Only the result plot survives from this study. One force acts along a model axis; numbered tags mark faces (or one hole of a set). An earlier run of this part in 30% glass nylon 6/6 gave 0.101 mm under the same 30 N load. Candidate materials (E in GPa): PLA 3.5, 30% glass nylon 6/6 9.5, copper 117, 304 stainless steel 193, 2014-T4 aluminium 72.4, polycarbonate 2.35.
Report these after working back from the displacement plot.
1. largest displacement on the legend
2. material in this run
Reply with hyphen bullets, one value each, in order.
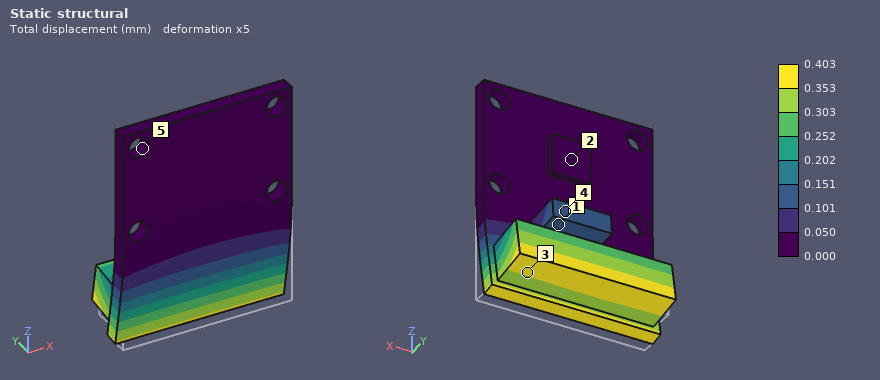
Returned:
- 0.403 mm
- polycarbonate
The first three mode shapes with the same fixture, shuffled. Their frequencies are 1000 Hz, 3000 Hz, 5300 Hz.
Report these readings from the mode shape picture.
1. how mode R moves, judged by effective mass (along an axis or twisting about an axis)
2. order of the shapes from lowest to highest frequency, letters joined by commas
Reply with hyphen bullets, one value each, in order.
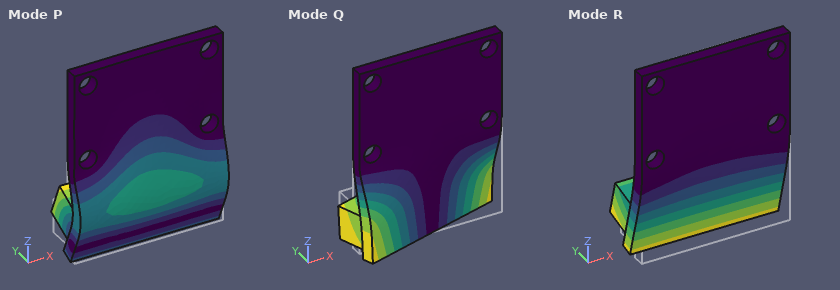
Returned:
- along Y
- R, Q, P
